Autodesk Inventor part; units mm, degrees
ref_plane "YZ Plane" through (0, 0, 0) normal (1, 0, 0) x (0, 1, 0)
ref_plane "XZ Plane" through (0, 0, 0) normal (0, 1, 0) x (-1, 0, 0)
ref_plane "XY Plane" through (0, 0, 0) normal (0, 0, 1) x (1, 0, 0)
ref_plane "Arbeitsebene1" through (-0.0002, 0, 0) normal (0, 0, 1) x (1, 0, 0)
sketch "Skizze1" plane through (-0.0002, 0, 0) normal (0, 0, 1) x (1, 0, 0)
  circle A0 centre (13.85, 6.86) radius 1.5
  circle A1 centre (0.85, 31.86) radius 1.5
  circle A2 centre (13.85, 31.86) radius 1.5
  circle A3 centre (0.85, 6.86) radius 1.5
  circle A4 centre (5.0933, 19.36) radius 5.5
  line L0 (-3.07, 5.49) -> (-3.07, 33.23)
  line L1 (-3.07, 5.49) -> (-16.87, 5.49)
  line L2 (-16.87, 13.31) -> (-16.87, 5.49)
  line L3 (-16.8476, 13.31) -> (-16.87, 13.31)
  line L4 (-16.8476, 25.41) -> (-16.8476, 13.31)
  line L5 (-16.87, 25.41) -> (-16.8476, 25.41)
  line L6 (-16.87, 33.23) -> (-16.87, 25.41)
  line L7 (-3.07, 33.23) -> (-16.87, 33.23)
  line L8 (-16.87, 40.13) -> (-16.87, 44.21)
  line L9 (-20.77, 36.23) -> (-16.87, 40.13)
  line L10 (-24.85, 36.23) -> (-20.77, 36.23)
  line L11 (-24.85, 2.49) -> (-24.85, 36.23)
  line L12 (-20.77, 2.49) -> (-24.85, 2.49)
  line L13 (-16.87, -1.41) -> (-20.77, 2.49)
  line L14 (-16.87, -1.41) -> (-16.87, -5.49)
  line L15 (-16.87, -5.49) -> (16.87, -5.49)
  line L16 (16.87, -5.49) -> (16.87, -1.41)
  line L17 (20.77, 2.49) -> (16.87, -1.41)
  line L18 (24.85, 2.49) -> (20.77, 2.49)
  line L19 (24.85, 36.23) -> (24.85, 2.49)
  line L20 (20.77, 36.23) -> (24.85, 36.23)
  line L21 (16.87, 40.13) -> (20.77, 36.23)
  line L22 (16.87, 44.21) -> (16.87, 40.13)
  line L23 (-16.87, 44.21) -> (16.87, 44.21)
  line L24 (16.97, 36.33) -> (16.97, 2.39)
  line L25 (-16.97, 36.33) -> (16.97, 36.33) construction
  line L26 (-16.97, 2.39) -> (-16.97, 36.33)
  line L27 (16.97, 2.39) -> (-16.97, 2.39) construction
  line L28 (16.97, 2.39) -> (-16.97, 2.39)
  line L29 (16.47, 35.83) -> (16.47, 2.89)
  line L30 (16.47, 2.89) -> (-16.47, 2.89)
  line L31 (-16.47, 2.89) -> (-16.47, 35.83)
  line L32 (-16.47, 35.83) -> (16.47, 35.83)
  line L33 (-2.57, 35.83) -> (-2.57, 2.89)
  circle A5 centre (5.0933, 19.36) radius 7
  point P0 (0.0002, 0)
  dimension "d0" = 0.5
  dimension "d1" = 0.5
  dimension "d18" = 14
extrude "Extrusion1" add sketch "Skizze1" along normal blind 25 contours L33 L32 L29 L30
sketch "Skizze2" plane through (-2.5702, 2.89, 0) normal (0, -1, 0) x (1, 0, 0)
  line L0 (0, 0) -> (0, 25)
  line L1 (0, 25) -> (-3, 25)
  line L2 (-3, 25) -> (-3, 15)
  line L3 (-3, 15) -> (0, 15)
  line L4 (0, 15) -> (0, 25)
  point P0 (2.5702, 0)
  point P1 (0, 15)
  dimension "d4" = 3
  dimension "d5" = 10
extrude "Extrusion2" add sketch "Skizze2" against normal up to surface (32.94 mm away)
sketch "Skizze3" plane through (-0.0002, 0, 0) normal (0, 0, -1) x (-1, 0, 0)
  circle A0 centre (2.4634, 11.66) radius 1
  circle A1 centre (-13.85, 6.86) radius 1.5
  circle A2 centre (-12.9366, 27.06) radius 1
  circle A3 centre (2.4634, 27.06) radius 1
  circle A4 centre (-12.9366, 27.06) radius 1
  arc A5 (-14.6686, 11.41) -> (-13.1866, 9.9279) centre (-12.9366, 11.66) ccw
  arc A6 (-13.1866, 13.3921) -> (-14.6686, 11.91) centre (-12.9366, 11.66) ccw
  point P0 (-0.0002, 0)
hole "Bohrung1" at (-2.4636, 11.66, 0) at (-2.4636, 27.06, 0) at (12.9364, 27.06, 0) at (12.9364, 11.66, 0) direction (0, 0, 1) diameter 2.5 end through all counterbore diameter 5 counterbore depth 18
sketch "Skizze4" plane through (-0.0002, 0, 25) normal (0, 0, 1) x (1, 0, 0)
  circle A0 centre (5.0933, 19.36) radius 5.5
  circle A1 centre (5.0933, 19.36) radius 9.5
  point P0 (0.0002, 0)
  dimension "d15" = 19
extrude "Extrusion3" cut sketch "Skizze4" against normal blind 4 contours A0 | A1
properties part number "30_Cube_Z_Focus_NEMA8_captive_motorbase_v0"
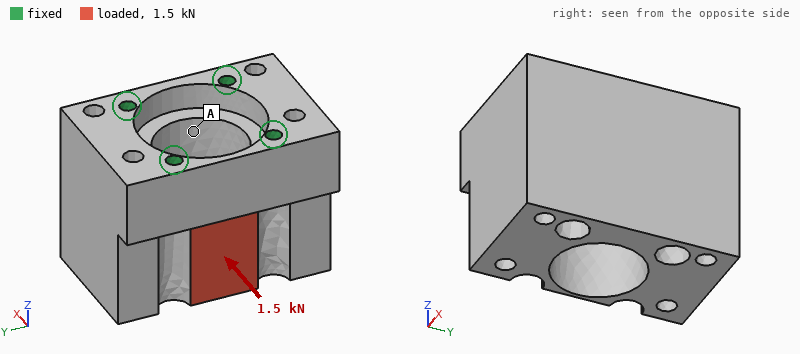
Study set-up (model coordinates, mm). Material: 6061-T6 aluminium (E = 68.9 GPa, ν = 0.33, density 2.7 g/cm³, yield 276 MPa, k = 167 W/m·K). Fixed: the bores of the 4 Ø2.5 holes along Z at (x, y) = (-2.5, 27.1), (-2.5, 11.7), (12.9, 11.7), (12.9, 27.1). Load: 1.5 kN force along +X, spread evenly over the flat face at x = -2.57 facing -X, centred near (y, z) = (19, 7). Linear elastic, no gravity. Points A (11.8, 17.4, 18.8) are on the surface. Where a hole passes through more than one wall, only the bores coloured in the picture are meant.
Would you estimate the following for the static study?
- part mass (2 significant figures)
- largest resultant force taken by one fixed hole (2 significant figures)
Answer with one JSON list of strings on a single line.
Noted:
["28 g", "800 N"]
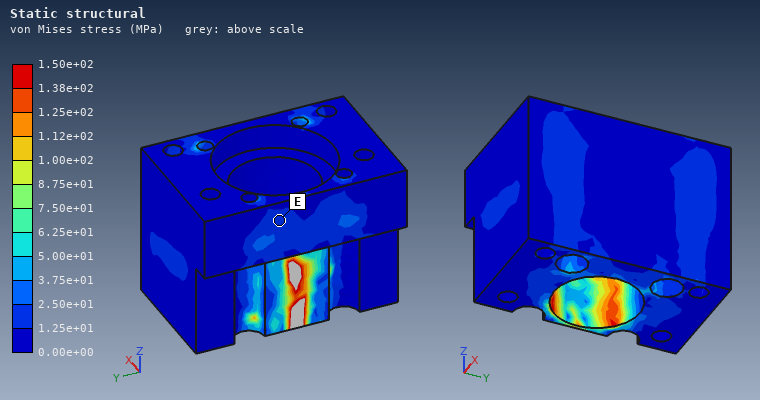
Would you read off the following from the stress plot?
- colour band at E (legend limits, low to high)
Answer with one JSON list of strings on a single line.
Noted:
["1.25e+01 to 2.50e+01 MPa"]
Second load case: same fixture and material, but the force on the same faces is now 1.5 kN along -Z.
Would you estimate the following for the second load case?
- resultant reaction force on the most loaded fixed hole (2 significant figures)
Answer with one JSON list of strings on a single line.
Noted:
["760 N"]
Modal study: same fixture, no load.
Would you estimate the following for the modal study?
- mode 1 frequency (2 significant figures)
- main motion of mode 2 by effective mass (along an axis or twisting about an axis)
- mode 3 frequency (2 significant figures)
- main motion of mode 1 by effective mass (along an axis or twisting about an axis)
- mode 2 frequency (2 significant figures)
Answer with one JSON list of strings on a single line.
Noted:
["16 kHz", "along X", "23 kHz", "along Y", "19 kHz"]
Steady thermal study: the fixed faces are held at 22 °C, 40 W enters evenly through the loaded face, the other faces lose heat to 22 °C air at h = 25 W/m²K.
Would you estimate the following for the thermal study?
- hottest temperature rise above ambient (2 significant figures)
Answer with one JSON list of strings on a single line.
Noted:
["44 K"]
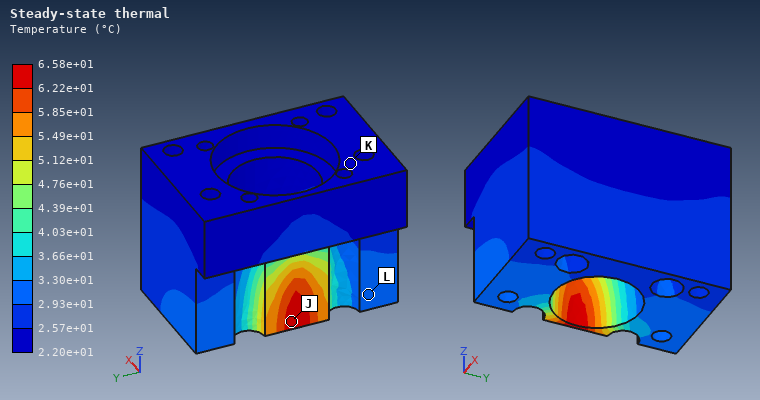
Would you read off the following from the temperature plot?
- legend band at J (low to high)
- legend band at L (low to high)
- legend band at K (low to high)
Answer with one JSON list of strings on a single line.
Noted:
["6.22e+01 to 6.58e+01 °C", "2.93e+01 to 3.30e+01 °C", "2.20e+01 to 2.57e+01 °C"]
